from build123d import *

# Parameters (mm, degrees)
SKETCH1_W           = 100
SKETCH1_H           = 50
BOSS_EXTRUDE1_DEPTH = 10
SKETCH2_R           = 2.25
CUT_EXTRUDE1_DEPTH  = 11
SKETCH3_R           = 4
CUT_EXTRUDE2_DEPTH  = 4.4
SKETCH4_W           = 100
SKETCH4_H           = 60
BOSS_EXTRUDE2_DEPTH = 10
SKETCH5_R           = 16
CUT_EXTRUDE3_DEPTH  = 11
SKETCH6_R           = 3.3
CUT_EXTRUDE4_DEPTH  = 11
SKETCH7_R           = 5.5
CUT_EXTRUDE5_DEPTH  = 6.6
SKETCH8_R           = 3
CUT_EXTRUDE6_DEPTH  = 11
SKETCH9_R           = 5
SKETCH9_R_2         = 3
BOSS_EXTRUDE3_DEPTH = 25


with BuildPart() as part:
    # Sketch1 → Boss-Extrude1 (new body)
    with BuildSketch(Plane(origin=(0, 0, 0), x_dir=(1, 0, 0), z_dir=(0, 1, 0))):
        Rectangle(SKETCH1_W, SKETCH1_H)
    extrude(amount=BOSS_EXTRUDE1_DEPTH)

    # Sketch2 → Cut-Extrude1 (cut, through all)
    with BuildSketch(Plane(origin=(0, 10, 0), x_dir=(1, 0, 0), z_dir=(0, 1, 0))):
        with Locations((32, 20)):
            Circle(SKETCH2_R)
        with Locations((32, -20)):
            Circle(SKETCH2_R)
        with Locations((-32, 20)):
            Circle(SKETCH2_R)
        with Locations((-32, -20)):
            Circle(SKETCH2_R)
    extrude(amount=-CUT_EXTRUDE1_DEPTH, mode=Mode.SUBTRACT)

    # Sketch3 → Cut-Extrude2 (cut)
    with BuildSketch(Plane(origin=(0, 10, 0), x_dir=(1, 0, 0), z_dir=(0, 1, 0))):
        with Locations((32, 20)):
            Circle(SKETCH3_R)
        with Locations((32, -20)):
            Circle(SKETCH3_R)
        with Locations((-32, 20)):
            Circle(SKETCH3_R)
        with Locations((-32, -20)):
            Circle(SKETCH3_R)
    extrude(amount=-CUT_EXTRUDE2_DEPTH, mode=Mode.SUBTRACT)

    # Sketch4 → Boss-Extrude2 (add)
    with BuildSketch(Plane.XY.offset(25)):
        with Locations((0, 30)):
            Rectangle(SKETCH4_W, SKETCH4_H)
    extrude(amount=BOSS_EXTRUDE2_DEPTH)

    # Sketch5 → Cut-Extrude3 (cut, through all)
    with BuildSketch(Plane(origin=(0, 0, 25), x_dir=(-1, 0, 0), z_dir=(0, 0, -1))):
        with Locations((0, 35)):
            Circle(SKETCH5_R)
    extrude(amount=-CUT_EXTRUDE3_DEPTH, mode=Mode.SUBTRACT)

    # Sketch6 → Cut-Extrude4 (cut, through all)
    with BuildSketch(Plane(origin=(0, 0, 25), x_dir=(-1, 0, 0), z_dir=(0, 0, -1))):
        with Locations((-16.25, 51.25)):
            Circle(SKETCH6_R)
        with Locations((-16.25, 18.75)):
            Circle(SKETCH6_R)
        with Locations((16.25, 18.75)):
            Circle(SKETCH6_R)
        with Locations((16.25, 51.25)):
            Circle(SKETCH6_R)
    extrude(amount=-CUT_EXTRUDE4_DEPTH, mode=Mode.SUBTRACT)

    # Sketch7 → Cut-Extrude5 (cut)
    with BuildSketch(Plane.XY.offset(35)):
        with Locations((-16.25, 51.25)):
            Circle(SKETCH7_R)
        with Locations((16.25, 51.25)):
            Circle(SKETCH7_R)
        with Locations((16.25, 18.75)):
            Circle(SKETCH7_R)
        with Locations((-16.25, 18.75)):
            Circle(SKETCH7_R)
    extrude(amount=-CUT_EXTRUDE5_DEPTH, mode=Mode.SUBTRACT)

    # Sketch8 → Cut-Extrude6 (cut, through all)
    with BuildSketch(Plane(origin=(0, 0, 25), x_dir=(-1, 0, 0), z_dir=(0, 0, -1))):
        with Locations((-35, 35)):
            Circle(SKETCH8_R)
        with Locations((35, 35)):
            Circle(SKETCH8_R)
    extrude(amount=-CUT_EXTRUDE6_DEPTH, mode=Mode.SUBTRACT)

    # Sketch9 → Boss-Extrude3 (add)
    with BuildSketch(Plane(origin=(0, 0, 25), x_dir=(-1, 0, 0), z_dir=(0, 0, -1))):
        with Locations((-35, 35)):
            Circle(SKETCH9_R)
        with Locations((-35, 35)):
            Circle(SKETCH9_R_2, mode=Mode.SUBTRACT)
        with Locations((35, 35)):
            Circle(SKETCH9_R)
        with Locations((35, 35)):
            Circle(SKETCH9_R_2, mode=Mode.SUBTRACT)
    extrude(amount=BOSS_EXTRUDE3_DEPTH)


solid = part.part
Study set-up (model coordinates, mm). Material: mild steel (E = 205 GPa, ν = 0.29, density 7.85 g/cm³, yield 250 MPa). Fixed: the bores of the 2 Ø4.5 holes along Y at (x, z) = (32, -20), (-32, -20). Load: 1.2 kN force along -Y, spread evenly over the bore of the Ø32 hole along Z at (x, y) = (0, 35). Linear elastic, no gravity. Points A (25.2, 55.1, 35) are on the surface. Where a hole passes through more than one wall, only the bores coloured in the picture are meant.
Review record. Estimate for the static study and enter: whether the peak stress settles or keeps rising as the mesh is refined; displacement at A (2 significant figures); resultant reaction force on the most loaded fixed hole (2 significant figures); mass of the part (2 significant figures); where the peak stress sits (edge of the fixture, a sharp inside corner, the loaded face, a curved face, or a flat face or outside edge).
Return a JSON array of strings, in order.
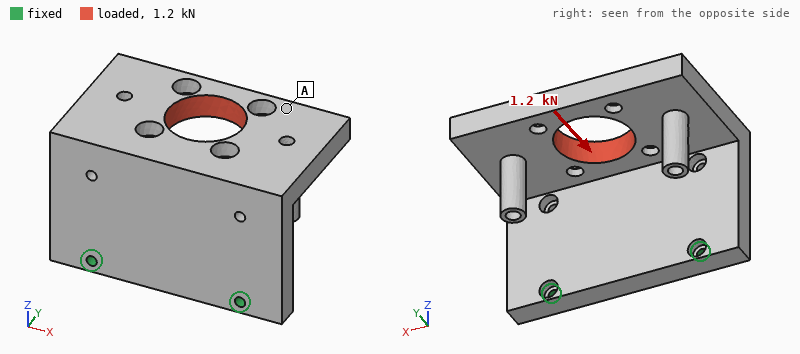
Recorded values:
["keeps rising", "0.17 mm", "600 N", "780 g", "edge of the fixture"]
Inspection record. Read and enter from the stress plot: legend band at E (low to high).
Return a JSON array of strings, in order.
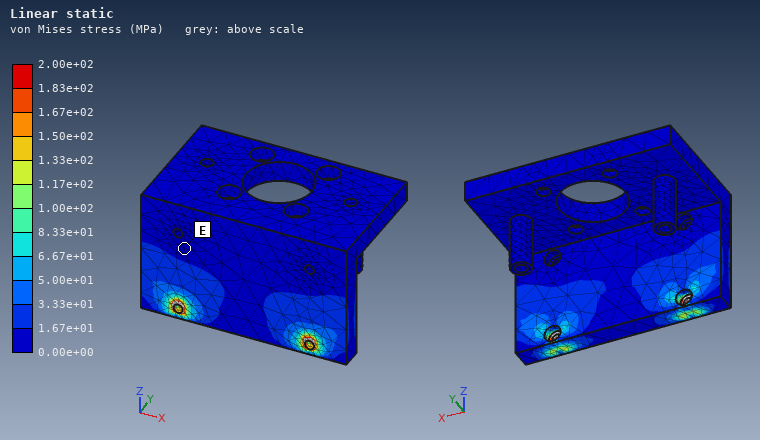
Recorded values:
["0.00e+00 to 1.67e+01 MPa"]
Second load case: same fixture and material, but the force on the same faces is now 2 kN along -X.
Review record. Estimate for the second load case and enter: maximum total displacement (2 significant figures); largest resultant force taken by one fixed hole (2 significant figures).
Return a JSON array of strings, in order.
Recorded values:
["61 µm", "2.0 kN"]
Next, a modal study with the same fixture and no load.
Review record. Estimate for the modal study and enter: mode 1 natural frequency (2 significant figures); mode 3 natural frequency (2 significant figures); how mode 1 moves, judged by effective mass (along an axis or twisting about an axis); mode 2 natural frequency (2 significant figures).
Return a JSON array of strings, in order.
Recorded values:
["660 Hz", "2200 Hz", "along Y", "1500 Hz"]
